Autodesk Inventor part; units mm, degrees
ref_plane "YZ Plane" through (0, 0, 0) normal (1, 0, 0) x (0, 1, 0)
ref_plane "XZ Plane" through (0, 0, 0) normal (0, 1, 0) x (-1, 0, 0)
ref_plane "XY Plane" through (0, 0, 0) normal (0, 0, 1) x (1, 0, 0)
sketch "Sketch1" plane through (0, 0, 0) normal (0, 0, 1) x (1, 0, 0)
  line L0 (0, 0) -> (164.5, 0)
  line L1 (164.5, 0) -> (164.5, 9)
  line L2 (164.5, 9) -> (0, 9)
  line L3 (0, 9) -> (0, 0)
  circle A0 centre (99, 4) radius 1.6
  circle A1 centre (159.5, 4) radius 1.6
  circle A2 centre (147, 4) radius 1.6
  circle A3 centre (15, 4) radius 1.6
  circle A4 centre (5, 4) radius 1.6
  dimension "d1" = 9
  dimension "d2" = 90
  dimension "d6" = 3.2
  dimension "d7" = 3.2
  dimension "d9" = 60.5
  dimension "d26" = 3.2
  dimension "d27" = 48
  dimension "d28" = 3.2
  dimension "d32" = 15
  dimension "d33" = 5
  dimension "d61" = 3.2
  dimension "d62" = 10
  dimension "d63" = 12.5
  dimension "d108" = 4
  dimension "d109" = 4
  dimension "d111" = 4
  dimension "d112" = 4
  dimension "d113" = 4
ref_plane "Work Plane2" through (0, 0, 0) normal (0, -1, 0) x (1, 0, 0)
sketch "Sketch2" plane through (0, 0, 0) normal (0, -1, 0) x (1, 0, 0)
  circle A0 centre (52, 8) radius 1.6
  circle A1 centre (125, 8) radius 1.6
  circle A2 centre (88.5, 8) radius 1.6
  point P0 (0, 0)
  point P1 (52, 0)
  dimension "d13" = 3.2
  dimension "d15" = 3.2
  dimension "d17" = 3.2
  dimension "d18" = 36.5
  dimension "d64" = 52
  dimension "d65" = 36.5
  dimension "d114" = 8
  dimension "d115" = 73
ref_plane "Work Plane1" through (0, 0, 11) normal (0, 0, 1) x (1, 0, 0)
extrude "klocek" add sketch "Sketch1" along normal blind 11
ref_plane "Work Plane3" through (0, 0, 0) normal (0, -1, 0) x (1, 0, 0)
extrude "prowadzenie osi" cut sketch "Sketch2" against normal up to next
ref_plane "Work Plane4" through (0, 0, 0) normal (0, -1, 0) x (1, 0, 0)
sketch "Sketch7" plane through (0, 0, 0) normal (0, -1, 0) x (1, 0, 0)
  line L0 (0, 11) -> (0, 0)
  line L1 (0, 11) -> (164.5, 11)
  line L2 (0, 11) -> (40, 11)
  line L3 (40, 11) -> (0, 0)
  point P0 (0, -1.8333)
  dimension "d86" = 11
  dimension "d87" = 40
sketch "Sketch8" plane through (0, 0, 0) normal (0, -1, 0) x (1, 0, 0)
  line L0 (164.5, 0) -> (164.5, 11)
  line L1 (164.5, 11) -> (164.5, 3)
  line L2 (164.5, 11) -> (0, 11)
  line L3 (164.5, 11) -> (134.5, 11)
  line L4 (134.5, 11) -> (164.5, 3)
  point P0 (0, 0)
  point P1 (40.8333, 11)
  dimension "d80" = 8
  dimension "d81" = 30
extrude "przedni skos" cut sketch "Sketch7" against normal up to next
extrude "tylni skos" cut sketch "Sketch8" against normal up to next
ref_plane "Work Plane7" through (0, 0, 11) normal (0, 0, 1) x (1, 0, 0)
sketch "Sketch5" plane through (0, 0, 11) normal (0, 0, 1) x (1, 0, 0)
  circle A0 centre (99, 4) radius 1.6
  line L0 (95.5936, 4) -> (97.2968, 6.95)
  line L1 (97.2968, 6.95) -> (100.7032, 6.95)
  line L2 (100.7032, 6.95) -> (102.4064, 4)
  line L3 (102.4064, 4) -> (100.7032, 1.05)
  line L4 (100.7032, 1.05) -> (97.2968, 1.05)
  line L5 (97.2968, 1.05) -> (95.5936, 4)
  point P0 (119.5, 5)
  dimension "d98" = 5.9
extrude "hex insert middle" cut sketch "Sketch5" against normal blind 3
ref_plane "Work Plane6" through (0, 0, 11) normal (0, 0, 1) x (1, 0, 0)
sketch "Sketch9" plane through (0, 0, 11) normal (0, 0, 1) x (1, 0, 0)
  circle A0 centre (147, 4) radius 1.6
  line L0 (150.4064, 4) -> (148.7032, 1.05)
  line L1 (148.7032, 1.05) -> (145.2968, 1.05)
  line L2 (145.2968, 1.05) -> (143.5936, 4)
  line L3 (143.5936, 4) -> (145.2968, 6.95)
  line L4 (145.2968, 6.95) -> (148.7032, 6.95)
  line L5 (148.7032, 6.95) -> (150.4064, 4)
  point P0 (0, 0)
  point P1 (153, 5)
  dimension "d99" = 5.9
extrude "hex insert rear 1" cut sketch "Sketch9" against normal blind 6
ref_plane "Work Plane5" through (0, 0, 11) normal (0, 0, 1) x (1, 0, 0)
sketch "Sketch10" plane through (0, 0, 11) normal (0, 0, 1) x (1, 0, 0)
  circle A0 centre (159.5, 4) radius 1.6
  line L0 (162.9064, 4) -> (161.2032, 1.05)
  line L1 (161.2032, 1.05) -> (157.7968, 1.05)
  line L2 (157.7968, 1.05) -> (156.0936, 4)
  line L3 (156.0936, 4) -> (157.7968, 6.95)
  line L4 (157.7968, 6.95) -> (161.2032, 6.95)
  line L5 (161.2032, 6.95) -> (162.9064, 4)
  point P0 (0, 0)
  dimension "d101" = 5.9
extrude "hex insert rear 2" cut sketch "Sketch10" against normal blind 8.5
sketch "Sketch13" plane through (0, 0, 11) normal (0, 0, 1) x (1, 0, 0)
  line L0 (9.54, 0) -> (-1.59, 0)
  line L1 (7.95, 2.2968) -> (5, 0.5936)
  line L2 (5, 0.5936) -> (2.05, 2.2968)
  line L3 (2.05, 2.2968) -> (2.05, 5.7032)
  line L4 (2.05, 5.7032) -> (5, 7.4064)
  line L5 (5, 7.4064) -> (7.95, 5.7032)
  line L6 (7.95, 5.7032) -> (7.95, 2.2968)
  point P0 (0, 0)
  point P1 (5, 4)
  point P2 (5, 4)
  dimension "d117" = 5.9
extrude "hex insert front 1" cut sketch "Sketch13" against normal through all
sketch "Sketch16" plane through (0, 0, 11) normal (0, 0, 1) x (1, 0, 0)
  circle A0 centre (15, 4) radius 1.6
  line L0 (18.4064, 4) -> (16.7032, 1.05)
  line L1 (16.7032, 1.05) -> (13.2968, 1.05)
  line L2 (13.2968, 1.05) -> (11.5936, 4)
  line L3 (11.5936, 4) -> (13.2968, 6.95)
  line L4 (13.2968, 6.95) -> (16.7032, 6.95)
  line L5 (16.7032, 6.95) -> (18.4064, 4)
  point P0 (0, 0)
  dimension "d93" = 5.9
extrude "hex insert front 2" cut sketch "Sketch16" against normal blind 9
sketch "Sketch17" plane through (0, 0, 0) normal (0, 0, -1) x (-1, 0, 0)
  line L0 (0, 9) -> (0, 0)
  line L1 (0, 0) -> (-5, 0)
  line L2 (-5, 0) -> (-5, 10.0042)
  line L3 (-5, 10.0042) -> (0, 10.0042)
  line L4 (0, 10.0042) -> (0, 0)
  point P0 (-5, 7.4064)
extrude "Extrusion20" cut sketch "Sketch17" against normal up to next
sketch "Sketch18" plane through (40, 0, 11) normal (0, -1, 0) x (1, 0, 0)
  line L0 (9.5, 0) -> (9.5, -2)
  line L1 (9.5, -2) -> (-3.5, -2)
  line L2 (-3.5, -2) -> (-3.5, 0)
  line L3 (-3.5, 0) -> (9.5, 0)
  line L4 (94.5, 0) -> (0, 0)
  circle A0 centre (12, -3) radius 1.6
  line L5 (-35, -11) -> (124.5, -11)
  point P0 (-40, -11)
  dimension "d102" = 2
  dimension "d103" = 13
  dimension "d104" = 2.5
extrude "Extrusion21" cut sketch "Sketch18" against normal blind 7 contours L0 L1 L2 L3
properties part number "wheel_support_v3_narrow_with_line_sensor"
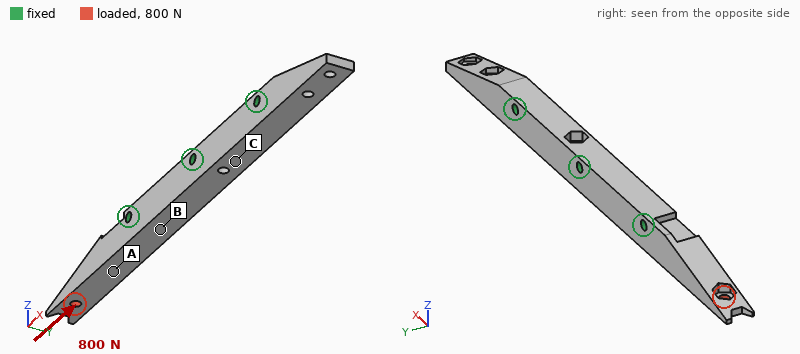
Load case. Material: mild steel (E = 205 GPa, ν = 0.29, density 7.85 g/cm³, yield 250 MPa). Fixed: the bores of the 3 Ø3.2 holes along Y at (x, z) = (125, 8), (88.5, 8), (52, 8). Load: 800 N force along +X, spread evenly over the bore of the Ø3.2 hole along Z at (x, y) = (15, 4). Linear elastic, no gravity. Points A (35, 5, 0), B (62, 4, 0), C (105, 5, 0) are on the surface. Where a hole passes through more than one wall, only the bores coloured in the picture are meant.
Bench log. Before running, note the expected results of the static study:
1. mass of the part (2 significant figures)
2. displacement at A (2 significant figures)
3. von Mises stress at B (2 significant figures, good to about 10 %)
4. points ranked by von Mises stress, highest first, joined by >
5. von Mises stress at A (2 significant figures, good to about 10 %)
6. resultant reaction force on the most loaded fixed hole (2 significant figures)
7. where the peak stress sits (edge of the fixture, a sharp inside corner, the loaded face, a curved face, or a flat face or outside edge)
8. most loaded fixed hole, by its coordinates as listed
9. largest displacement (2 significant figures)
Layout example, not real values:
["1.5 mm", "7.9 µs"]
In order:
["97 g", "6.5 µm", "11 MPa", "A > B > C", "32 MPa", "570 N", "the loaded face", "(52, 8)", "39 µm"]
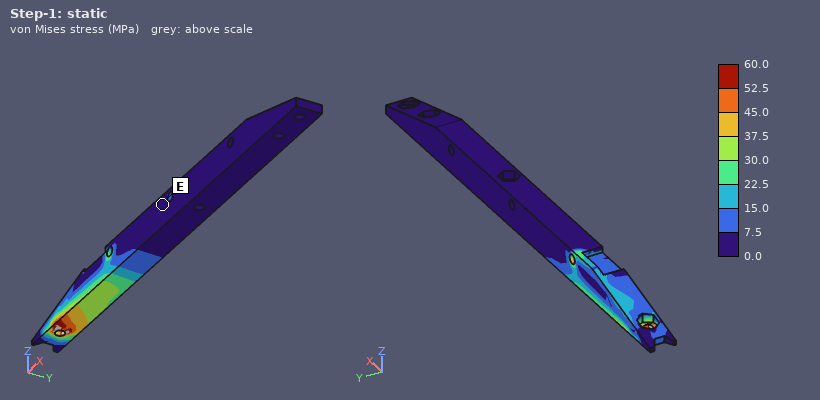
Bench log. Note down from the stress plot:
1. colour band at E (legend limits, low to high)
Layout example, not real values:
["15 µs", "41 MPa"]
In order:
["0.0 to 7.5 MPa"]
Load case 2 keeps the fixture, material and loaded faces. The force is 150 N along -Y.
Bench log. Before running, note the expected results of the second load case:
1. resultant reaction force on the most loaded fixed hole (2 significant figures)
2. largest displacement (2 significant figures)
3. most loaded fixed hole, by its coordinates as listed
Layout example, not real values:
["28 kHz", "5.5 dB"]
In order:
["180 N", "35 µm", "(52, 8)"]
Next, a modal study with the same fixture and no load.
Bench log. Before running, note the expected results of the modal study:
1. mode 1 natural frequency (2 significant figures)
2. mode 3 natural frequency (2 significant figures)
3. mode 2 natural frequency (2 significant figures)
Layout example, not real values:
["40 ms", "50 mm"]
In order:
["4900 Hz", "6600 Hz", "5400 Hz"]
